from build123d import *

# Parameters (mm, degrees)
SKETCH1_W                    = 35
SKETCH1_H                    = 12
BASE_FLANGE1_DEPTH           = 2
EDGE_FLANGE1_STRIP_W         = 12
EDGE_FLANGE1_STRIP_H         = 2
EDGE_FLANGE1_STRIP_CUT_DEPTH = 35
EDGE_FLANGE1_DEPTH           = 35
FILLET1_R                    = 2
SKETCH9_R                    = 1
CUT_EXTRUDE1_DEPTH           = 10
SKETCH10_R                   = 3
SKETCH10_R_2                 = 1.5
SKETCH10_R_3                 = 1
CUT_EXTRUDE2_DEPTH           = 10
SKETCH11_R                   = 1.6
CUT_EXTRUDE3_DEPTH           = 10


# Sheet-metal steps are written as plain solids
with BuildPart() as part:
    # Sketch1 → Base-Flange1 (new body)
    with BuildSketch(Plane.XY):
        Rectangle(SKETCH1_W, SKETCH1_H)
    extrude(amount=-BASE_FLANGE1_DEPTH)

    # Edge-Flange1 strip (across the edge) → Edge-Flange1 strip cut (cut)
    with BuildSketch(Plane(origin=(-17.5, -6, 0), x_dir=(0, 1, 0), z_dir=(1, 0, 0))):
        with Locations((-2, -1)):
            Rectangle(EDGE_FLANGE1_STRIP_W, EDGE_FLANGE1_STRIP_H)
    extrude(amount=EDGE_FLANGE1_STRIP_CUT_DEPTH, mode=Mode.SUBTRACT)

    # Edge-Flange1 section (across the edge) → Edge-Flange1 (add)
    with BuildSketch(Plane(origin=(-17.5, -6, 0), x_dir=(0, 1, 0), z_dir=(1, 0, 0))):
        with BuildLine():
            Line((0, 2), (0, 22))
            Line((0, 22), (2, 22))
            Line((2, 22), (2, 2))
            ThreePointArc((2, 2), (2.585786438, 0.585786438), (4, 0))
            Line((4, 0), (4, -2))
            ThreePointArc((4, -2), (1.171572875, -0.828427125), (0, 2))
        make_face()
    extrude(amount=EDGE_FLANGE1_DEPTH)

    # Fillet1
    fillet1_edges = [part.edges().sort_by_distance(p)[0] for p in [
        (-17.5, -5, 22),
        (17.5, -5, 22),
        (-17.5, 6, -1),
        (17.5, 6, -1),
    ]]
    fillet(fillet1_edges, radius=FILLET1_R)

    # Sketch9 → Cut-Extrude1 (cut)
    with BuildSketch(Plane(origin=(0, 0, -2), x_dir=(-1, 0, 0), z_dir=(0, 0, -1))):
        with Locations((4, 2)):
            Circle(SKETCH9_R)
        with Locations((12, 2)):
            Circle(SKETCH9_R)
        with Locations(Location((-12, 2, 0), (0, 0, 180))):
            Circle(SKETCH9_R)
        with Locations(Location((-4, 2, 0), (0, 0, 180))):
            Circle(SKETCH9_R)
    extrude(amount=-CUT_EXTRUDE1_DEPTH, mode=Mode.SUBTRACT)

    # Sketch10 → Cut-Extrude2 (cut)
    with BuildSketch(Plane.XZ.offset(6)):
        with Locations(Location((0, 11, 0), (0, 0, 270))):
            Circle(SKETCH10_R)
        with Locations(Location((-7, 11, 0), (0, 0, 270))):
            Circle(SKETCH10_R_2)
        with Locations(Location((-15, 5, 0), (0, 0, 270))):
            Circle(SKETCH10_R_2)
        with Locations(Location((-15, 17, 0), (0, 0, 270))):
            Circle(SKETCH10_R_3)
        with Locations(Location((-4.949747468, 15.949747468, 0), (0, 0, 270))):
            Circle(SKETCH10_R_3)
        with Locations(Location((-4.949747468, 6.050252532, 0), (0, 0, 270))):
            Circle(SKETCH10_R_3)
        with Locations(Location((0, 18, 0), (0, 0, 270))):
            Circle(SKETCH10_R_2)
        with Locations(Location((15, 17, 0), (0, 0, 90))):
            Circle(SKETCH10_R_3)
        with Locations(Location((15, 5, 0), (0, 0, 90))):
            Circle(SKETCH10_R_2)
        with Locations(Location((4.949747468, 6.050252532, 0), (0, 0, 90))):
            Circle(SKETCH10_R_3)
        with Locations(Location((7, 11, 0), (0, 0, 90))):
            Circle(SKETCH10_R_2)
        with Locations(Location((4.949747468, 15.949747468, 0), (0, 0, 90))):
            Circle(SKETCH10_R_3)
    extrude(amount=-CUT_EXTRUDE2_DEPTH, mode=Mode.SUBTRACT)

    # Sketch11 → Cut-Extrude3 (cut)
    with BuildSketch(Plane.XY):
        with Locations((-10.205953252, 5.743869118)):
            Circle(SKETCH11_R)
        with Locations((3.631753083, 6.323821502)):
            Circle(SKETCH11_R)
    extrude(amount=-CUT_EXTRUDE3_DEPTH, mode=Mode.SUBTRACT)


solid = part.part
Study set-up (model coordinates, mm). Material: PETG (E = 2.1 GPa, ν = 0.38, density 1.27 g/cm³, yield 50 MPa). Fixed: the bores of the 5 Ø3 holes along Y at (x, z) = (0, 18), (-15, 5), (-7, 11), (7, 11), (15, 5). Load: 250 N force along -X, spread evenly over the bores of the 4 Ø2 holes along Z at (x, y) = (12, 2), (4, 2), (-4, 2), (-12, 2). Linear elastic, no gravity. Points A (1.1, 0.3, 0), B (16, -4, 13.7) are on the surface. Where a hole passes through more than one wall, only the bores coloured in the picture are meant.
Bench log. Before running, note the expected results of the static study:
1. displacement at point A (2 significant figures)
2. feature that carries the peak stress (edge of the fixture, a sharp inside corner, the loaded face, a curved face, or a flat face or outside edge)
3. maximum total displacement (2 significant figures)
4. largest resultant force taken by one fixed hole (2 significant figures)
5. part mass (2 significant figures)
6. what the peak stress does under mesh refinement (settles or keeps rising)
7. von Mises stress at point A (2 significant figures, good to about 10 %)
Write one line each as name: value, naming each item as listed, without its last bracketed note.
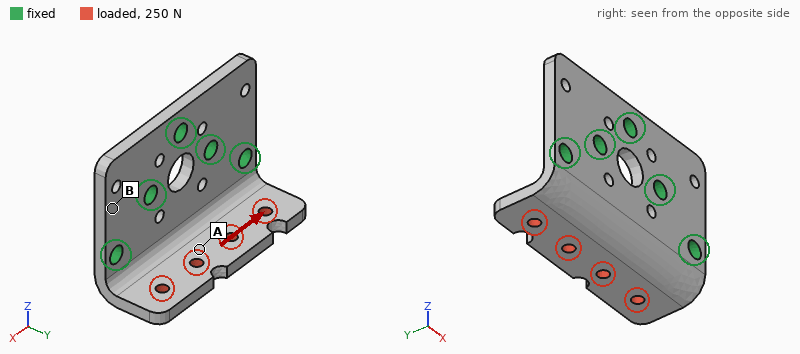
displacement at point A: 0.12 mm
feature that carries the peak stress: edge of the fixture
maximum total displacement: 0.43 mm
largest resultant force taken by one fixed hole: 120 N
part mass: 2.6 g
what the peak stress does under mesh refinement: keeps rising
von Mises stress at point A: 12 MPa
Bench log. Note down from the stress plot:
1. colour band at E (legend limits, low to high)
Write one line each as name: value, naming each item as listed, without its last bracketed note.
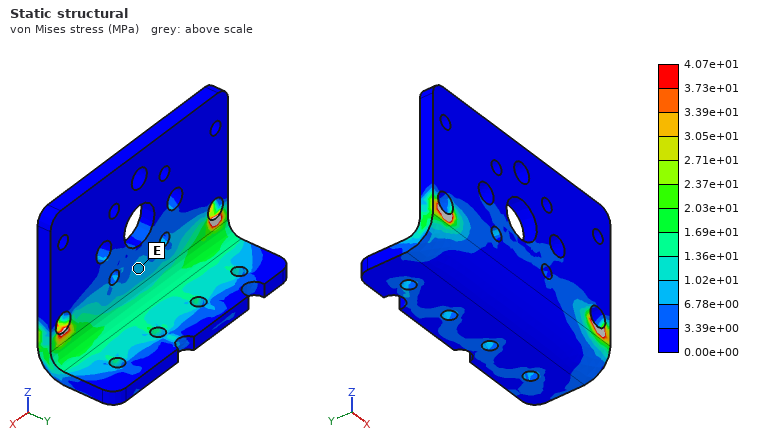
colour band at E: 6.78e+00 to 1.02e+01 MPa
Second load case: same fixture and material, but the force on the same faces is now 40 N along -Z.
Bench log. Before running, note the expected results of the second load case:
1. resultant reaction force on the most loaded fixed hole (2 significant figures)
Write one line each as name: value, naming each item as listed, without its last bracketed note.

resultant reaction force on the most loaded fixed hole: 19 N
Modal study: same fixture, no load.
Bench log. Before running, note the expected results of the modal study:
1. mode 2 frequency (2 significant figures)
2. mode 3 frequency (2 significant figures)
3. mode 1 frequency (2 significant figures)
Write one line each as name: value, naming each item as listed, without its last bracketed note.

mode 2 frequency: 3000 Hz
mode 3 frequency: 3700 Hz
mode 1 frequency: 2100 Hz
